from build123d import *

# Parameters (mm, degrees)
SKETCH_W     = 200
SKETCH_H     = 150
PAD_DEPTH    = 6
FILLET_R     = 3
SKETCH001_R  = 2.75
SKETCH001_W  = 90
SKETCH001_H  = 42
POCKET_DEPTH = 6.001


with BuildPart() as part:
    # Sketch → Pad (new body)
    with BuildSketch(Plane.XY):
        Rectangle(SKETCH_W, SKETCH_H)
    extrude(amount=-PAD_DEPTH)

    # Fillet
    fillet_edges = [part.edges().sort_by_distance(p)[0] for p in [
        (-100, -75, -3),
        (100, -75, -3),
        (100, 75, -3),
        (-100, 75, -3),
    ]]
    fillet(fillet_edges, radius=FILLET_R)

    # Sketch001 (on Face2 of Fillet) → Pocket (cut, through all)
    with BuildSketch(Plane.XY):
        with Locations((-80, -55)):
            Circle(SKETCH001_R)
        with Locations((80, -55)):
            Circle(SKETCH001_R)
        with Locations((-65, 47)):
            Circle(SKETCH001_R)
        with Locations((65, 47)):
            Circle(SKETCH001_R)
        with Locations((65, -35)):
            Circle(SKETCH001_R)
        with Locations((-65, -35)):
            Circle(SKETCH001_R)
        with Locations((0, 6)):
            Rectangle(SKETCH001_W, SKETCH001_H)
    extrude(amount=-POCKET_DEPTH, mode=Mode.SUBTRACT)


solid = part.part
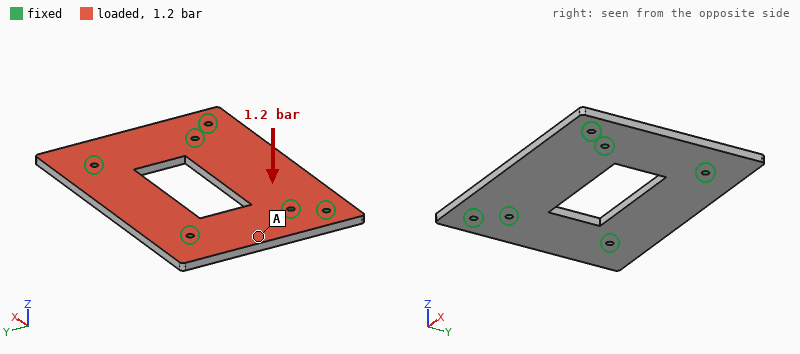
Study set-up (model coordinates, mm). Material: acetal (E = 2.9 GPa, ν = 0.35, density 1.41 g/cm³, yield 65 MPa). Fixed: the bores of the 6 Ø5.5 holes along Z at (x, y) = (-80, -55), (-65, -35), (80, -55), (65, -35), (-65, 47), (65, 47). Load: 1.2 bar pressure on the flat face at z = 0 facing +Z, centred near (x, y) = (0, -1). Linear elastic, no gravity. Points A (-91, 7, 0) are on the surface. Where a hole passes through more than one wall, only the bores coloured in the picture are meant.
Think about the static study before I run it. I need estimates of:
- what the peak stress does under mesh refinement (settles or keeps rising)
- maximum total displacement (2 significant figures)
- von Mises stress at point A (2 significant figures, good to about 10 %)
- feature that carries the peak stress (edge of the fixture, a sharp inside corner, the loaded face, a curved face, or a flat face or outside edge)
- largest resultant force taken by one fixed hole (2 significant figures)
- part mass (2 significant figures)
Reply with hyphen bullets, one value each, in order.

- keeps rising
- 2.7 mm
- 4.4 MPa
- edge of the fixture
- 710 N
- 220 g
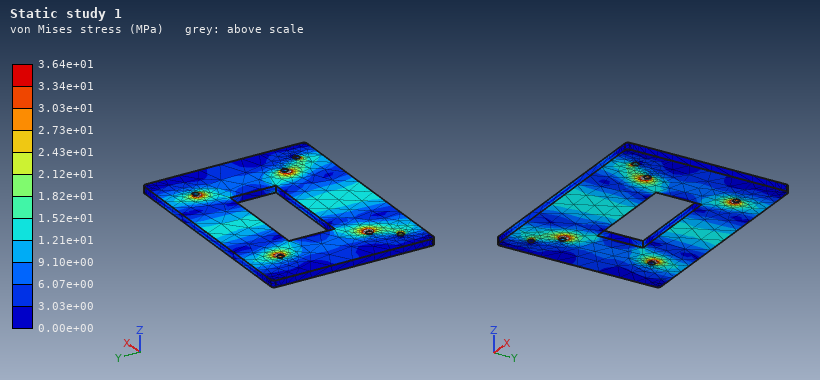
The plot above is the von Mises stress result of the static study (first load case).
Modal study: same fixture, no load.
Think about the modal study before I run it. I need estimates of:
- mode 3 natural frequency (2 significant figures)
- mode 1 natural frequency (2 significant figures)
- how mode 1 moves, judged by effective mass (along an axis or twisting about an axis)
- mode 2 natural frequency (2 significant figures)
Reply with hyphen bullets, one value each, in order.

- 740 Hz
- 450 Hz
- along Z
- 480 Hz
